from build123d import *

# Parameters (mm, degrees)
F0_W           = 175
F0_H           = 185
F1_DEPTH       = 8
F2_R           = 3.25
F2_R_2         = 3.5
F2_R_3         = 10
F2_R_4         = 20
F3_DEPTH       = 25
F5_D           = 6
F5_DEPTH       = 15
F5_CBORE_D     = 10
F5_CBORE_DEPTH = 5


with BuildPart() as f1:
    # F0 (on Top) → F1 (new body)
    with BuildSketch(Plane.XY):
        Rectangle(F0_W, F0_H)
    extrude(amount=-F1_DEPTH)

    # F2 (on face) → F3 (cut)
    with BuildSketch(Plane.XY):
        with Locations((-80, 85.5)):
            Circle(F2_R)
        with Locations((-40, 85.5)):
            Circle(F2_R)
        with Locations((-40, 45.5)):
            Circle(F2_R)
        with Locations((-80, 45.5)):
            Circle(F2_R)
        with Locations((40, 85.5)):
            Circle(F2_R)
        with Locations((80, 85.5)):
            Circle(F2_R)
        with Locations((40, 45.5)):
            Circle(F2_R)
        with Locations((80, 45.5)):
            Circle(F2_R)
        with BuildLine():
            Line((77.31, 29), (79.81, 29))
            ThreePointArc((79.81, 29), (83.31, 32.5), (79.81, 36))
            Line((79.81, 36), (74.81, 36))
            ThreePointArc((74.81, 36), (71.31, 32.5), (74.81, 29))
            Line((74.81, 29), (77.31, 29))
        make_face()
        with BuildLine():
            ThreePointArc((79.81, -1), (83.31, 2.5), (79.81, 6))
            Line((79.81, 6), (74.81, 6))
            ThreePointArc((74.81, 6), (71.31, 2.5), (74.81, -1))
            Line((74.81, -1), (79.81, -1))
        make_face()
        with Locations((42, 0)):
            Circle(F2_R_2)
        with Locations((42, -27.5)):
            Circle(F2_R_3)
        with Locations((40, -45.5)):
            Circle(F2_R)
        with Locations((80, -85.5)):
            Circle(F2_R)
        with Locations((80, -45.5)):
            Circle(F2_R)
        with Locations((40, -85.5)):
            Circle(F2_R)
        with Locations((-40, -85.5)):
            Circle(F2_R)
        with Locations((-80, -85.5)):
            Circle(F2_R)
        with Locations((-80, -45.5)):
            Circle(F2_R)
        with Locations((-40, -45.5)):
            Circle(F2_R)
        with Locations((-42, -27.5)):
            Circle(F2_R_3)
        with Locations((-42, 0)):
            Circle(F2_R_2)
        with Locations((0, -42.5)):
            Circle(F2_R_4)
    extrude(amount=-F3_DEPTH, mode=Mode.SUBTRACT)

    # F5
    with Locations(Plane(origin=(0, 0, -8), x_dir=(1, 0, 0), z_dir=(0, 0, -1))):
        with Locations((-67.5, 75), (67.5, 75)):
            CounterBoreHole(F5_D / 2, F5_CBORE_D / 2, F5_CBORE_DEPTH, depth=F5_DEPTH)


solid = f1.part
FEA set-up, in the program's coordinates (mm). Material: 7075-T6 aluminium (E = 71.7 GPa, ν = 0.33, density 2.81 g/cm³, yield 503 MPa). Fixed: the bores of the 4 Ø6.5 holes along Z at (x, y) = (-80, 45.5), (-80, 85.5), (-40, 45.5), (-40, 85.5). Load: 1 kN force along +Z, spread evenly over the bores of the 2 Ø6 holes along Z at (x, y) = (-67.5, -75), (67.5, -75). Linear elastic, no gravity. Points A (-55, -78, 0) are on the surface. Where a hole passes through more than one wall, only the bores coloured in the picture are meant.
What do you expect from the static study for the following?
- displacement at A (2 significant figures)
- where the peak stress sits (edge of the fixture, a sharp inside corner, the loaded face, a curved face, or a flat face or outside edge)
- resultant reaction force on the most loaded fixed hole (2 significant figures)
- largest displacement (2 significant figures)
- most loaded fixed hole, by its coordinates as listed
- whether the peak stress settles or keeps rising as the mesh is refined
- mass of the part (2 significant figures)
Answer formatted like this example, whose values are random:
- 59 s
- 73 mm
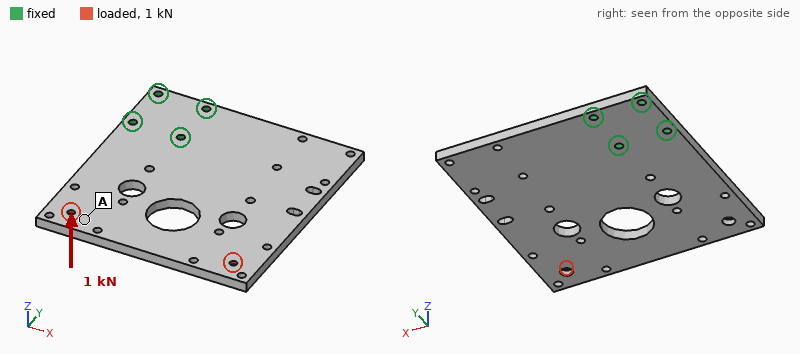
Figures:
- 1.6 mm
- edge of the fixture
- 3.1 kN
- 2.9 mm
- (-40, 45.5)
- keeps rising
- 670 g
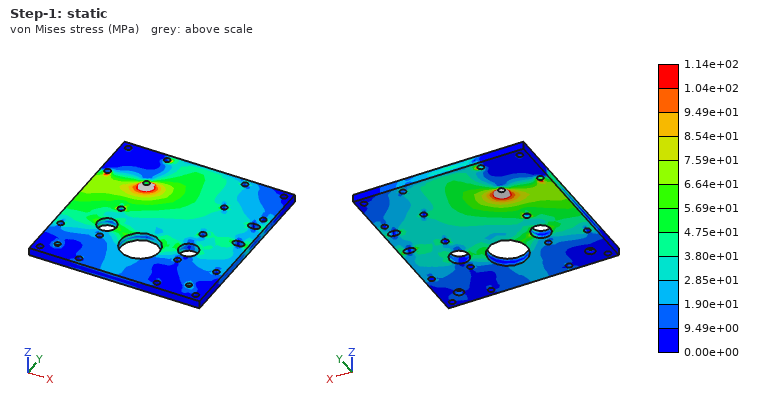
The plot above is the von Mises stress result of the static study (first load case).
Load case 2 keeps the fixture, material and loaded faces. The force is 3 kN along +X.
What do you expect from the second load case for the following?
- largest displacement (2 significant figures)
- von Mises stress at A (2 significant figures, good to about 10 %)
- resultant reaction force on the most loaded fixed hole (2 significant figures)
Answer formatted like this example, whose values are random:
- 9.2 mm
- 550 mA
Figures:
- 0.24 mm
- 11 MPa
- 5.6 kN
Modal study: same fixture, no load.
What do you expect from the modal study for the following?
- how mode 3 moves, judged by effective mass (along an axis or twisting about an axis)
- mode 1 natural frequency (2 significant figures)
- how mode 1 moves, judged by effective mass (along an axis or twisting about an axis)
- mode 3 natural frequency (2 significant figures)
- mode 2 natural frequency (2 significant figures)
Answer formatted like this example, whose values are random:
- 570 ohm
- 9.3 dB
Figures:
- along Z
- 240 Hz
- along Z
- 740 Hz
- 390 Hz
